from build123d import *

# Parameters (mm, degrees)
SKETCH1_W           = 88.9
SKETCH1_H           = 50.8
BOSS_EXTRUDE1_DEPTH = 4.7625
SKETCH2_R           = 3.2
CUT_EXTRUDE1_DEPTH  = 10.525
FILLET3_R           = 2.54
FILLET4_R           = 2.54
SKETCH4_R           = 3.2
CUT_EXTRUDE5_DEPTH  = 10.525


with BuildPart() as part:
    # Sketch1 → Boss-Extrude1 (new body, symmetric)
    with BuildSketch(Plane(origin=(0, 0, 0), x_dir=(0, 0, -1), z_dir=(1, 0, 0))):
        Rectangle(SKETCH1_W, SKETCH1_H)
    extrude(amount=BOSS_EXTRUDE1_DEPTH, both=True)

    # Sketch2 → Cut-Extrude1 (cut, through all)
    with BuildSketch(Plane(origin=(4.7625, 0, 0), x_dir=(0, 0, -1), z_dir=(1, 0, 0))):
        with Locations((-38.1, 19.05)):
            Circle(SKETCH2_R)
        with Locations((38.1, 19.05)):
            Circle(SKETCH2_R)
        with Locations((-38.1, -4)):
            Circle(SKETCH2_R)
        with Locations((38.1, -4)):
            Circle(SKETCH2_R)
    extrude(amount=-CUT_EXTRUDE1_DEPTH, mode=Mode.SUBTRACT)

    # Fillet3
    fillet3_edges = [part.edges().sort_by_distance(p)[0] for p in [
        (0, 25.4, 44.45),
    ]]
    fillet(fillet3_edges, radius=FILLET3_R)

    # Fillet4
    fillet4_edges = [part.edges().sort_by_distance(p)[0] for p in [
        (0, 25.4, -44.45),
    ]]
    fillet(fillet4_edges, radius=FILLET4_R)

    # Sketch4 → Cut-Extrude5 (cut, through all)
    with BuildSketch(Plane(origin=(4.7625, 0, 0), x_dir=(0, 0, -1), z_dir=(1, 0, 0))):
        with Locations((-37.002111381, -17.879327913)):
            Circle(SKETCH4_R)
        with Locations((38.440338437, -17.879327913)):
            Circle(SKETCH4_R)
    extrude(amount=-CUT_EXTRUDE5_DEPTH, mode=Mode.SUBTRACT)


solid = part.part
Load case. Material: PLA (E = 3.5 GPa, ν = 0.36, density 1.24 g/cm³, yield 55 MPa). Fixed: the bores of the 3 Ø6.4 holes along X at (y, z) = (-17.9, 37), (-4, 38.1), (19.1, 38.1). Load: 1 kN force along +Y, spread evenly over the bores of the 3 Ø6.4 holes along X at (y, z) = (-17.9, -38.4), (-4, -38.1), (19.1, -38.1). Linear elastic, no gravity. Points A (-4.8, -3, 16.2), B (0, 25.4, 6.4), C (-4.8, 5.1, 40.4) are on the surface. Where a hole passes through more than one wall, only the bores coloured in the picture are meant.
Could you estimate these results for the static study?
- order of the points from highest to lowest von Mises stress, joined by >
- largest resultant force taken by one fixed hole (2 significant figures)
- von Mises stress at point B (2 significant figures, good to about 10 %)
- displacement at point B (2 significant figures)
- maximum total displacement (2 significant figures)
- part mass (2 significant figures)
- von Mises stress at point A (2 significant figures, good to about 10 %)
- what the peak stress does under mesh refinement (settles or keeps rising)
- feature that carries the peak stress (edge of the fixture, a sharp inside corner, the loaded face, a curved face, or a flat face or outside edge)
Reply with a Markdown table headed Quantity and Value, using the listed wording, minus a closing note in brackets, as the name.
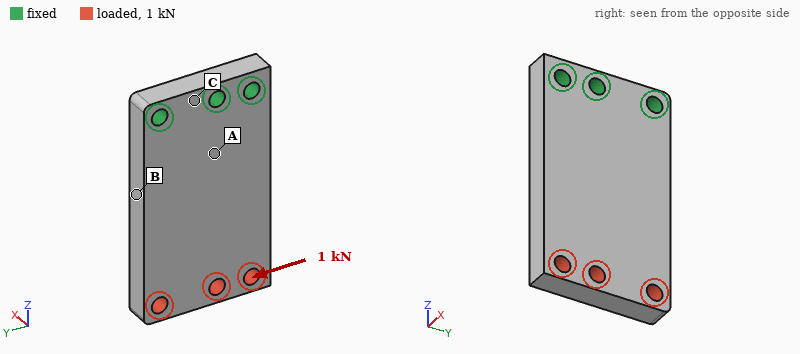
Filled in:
| Quantity | Value |
|---|---|
| order of the points from highest to lowest von Mises stress, joined by > | B > A > C |
| largest resultant force taken by one fixed hole | 2.0 kN |
| von Mises stress at point B | 11 MPa |
| displacement at point B | 0.20 mm |
| maximum total displacement | 0.63 mm |
| part mass | 51 g |
| von Mises stress at point A | 5.5 MPa |
| what the peak stress does under mesh refinement | keeps rising |
| feature that carries the peak stress | edge of the fixture |
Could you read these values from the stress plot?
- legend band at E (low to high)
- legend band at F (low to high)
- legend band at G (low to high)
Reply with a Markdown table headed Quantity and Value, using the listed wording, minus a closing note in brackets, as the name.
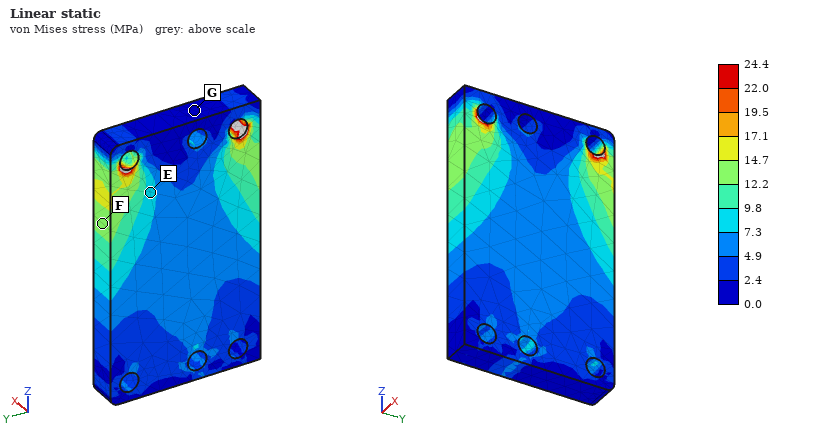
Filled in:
| Quantity | Value |
|---|---|
| legend band at E | 7.3 to 9.8 MPa |
| legend band at F | 12.2 to 14.7 MPa |
| legend band at G | 0.0 to 2.4 MPa |
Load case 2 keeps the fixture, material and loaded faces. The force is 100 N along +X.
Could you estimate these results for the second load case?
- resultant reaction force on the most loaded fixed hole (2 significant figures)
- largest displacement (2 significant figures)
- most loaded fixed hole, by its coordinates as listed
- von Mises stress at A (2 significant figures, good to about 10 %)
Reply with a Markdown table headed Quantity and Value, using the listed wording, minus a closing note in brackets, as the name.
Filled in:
| Quantity | Value |
|---|---|
| resultant reaction force on the most loaded fixed hole | 68 N |
| largest displacement | 1.2 mm |
| most loaded fixed hole, by its coordinates as listed | (-4, 38.1) |
| von Mises stress at A | 6.5 MPa |
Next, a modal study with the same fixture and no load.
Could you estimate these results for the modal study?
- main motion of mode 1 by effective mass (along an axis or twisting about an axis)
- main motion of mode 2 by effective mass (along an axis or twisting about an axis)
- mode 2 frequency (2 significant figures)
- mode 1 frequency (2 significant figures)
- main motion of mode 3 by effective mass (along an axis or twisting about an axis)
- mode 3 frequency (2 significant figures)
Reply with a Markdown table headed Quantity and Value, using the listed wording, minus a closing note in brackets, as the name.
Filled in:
| Quantity | Value |
|---|---|
| main motion of mode 1 by effective mass | along X |
| main motion of mode 2 by effective mass | twisting about Z |
| mode 2 frequency | 1300 Hz |
| mode 1 frequency | 410 Hz |
| main motion of mode 3 by effective mass | along Y |
| mode 3 frequency | 1700 Hz |
